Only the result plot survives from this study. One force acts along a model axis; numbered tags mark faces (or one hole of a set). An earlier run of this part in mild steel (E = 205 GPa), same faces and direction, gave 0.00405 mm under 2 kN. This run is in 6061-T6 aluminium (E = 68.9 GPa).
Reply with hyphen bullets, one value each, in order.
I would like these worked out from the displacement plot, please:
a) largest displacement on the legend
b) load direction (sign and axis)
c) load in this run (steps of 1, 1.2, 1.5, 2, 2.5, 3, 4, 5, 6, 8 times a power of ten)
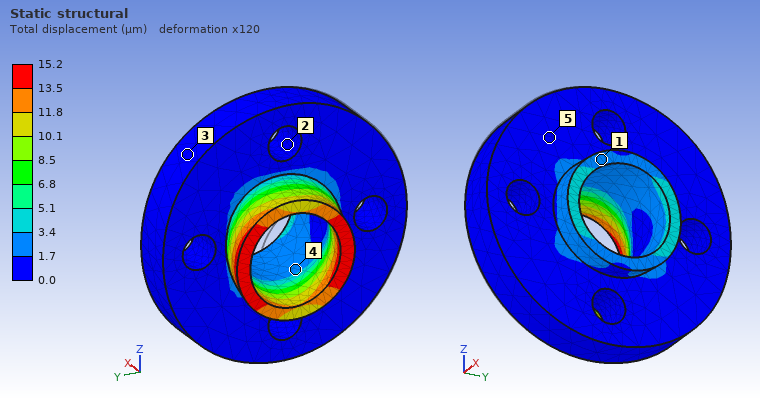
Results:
- 15.2 µm
- +Y
- 2.5 kN
